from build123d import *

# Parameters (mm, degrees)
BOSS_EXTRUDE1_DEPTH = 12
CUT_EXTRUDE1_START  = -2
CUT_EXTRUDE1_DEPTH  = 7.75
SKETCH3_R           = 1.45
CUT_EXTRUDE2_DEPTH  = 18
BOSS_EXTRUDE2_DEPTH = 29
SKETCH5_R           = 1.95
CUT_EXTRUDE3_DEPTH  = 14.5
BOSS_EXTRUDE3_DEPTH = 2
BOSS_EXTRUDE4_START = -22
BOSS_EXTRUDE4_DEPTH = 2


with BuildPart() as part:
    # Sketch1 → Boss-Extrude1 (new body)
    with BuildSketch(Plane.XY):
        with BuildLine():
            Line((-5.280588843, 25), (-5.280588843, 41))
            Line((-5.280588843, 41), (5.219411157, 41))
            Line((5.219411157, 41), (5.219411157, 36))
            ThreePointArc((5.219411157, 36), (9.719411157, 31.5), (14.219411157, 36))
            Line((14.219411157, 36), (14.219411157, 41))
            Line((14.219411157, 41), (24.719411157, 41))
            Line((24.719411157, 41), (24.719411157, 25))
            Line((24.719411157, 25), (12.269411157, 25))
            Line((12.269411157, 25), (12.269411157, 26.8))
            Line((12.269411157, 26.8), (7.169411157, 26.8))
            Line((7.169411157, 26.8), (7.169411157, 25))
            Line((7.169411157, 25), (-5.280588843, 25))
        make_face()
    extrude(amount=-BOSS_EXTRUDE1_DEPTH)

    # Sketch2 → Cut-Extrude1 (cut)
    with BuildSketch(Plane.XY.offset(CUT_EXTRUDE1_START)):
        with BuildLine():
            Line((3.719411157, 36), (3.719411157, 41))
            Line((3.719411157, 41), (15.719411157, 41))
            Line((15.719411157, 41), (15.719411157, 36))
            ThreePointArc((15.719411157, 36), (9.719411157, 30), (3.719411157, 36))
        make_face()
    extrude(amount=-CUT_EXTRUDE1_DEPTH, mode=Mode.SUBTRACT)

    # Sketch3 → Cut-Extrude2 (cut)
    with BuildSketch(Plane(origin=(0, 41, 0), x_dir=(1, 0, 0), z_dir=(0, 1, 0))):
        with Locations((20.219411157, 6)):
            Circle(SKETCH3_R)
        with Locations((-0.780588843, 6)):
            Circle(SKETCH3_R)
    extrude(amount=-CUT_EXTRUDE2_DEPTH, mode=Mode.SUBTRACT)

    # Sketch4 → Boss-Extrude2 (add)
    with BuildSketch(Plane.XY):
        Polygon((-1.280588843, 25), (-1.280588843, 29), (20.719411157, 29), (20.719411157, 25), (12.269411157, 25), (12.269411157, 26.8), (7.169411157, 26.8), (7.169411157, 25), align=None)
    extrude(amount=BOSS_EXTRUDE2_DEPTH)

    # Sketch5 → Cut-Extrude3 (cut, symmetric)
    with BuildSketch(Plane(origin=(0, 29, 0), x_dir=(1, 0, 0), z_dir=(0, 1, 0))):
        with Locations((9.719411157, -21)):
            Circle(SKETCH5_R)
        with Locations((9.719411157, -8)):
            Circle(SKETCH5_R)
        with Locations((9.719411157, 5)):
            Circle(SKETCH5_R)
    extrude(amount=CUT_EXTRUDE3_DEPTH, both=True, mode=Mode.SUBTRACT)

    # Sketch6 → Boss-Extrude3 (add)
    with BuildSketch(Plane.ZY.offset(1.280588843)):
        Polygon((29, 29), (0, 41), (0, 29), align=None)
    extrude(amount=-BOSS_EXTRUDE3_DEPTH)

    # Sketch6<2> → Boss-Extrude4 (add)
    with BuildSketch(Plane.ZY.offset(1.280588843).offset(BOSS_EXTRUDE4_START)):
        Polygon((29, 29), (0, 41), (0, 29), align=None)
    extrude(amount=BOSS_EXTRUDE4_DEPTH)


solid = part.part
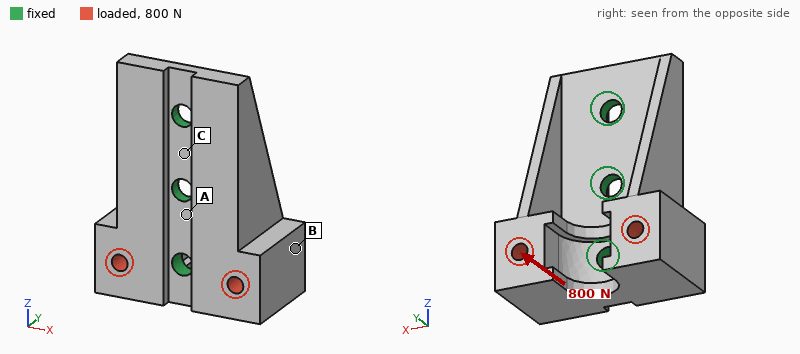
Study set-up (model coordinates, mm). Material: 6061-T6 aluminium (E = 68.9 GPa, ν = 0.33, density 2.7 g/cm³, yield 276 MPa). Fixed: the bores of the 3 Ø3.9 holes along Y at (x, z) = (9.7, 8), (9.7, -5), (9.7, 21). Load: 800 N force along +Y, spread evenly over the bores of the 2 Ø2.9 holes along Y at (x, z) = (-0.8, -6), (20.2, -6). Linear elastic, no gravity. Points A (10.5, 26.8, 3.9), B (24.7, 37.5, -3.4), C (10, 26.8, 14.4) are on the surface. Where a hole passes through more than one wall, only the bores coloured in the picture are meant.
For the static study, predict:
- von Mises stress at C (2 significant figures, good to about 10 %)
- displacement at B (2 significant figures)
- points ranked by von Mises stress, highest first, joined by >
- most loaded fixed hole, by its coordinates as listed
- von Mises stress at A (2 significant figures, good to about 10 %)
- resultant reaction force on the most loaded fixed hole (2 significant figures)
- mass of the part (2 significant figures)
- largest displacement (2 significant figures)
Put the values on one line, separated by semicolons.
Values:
15 MPa; 27 µm; A > C > B; (9.7, -5); 29 MPa; 770 N; 19 g; 33 µm
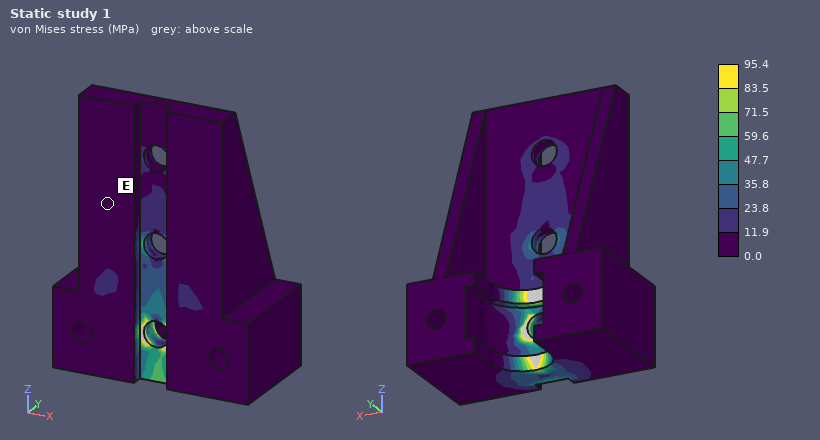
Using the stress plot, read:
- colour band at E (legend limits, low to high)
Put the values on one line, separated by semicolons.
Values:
0.0 to 11.9 MPa
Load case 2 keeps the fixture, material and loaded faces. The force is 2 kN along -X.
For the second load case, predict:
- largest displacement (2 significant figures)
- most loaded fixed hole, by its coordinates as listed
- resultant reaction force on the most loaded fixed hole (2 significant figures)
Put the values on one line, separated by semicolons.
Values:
63 µm; (9.7, -5); 2.1 kN
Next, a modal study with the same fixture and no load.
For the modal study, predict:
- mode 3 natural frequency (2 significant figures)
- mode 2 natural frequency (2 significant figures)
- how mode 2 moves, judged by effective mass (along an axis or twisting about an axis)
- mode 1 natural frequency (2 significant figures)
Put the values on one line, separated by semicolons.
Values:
13 kHz; 8900 Hz; along Y; 7100 Hz
